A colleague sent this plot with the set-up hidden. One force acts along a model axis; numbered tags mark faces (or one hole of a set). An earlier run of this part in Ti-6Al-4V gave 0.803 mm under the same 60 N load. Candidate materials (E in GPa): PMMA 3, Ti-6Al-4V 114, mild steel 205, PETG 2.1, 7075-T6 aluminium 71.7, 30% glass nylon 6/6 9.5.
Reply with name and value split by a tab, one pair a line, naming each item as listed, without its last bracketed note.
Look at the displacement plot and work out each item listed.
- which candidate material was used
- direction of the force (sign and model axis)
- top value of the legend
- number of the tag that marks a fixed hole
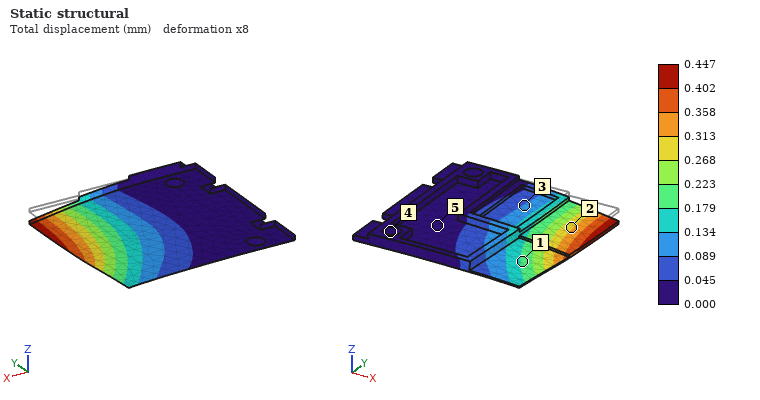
which candidate material was used	mild steel
direction of the force	-Z
top value of the legend	0.447 mm
number of the tag that marks a fixed hole	4
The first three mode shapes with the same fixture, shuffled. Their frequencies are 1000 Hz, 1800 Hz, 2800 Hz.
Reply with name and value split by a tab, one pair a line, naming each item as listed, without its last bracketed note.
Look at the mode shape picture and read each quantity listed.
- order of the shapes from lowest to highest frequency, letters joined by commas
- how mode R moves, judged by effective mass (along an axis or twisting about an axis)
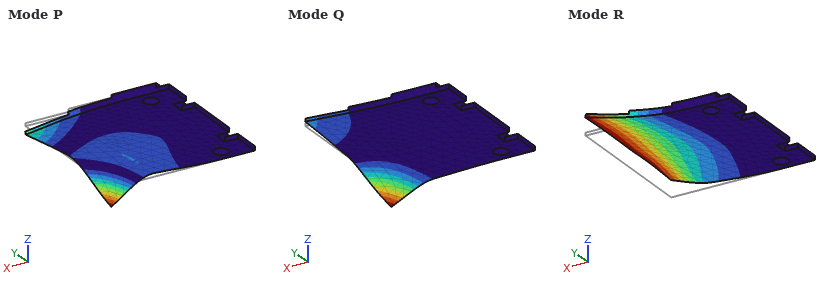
order of the shapes from lowest to highest frequency, letters joined by commas	R, Q, P
how mode R moves, judged by effective mass	along Z
